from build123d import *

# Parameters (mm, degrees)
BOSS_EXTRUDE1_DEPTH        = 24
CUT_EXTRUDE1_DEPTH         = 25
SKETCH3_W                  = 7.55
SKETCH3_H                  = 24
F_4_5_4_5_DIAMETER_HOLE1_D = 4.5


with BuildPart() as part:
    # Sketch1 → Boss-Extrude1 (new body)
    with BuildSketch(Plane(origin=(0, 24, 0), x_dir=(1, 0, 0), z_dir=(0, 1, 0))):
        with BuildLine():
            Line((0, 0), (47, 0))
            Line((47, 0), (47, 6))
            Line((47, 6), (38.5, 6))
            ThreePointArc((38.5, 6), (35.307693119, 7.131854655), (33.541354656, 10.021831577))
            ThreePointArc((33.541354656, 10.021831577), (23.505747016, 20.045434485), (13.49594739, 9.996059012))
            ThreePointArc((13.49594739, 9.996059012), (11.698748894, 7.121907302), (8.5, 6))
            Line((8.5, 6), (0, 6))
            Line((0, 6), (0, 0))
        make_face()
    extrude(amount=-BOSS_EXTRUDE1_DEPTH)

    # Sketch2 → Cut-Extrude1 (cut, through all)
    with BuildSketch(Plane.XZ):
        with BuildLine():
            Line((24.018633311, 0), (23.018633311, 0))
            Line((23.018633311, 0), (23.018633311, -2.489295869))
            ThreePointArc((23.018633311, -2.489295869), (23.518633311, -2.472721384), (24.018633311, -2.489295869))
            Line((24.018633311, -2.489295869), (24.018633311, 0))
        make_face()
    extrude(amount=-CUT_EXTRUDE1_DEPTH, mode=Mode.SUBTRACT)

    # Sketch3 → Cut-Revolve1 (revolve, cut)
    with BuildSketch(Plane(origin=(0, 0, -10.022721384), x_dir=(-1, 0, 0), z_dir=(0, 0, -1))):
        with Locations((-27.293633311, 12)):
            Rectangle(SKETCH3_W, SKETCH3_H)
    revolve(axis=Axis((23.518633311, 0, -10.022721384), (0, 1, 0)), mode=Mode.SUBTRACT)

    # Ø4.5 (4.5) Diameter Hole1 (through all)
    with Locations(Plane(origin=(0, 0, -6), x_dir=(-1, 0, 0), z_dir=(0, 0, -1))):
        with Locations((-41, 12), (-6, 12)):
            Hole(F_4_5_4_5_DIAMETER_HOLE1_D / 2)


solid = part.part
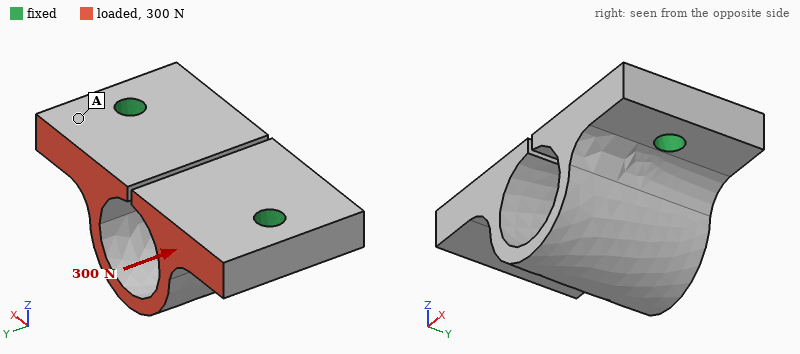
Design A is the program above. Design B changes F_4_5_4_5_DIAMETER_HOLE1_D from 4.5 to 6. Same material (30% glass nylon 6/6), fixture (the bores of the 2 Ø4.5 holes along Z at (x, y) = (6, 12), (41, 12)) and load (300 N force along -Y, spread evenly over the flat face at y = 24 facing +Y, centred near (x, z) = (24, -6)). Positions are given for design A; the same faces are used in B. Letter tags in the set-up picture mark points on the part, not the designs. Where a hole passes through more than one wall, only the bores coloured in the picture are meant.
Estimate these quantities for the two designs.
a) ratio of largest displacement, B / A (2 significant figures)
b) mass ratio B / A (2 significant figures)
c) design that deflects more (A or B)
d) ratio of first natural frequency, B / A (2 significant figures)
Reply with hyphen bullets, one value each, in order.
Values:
- 0.72
- 0.98
- A
- 1.2
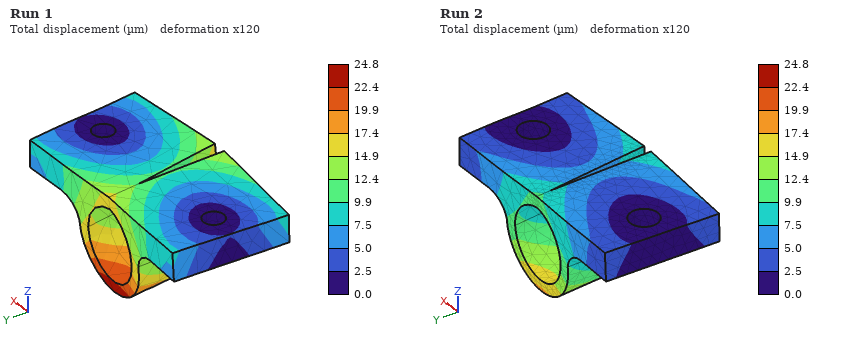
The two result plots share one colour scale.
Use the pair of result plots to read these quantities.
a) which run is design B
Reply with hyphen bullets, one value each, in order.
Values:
- Run 2
